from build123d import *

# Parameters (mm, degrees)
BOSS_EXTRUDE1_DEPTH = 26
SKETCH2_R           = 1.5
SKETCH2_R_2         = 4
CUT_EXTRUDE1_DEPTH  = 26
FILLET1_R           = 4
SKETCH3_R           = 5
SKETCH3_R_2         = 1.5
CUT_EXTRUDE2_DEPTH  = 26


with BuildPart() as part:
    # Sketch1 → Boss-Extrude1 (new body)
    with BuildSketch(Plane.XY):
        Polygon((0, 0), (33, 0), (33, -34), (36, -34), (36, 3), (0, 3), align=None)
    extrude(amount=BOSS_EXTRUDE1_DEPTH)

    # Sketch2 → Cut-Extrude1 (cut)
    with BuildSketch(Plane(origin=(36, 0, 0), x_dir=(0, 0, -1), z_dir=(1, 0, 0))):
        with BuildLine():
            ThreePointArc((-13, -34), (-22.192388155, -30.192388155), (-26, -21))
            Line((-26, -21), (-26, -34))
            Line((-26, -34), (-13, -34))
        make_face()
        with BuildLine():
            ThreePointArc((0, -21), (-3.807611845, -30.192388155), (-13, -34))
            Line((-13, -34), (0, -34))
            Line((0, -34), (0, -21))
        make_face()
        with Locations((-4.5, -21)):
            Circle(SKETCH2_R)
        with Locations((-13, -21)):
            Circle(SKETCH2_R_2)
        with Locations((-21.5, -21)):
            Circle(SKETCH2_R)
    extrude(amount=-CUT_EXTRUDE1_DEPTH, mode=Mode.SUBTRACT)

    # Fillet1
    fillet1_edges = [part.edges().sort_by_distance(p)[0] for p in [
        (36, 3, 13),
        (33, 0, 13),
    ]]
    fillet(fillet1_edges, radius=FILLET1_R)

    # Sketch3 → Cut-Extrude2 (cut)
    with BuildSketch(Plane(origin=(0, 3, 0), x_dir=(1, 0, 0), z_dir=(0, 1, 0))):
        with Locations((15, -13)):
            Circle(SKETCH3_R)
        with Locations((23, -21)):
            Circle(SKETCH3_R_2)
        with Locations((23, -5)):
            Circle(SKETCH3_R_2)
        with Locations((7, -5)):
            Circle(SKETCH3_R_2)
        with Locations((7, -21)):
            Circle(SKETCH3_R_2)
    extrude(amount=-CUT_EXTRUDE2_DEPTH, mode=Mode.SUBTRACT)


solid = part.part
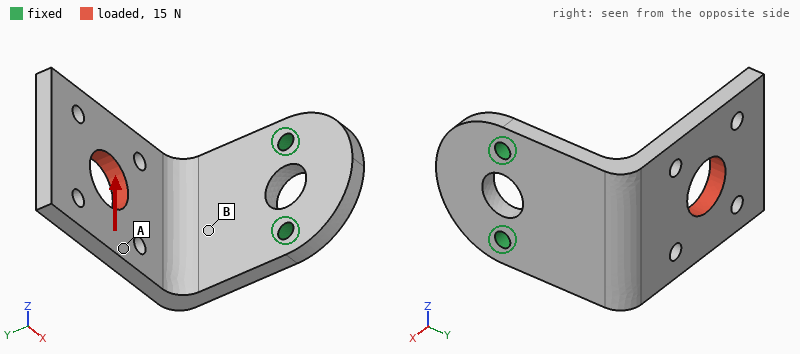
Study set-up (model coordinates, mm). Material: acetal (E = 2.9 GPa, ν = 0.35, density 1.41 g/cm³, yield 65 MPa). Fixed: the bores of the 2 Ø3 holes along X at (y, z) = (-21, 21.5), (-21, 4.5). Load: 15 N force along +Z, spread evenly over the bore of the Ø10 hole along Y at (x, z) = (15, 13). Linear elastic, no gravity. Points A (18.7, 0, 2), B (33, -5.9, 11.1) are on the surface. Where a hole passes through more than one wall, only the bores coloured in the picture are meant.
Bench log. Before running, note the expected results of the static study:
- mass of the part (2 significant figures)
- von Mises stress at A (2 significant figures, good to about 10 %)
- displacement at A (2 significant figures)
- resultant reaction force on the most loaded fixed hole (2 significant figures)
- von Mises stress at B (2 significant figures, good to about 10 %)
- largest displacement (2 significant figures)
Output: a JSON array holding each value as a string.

["6.7 g", "0.89 MPa", "0.29 mm", "24 N", "4.7 MPa", "0.54 mm"]
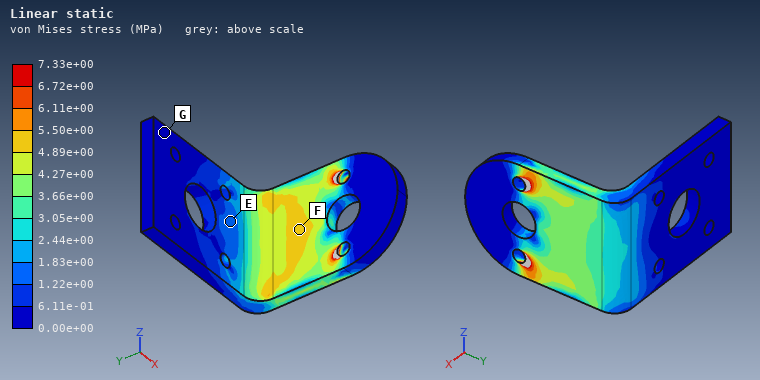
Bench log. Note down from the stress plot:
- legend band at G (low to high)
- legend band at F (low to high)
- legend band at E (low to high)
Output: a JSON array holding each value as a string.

["0.00e+00 to 6.11e-01 MPa", "4.89e+00 to 5.50e+00 MPa", "1.22e+00 to 1.83e+00 MPa"]
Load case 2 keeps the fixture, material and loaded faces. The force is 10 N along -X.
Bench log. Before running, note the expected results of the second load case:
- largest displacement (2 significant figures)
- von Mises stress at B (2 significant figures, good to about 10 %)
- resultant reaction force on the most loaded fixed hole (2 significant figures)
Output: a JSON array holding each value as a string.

["0.60 mm", "1.8 MPa", "5.0 N"]
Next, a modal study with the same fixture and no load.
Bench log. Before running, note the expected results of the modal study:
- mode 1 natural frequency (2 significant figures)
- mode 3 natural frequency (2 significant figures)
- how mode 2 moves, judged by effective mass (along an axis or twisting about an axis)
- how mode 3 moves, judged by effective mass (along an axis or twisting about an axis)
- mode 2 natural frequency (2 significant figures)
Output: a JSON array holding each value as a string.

["300 Hz", "910 Hz", "along Z", "along X", "570 Hz"]
